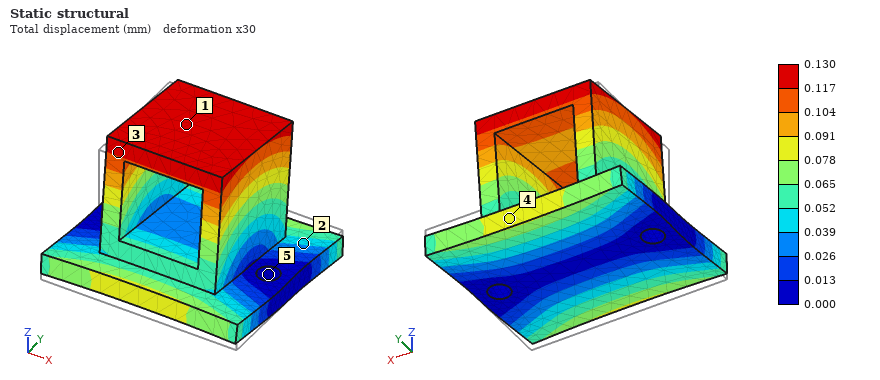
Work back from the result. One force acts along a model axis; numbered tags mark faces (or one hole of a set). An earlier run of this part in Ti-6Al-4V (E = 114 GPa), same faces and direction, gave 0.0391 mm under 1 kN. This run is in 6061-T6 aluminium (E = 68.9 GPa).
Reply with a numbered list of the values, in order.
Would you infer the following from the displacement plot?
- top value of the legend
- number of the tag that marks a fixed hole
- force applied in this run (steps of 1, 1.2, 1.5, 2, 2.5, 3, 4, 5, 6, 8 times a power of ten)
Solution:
1. 0.130 mm
2. 5
3. 2 kN
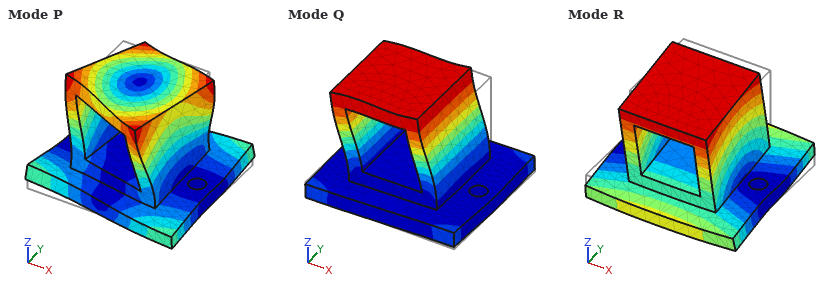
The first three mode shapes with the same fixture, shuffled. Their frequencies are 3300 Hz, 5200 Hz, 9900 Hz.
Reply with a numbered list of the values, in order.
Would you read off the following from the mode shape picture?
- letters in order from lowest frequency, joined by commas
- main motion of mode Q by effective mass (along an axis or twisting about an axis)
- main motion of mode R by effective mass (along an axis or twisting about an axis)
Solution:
1. R, Q, P
2. along X
3. along Y
